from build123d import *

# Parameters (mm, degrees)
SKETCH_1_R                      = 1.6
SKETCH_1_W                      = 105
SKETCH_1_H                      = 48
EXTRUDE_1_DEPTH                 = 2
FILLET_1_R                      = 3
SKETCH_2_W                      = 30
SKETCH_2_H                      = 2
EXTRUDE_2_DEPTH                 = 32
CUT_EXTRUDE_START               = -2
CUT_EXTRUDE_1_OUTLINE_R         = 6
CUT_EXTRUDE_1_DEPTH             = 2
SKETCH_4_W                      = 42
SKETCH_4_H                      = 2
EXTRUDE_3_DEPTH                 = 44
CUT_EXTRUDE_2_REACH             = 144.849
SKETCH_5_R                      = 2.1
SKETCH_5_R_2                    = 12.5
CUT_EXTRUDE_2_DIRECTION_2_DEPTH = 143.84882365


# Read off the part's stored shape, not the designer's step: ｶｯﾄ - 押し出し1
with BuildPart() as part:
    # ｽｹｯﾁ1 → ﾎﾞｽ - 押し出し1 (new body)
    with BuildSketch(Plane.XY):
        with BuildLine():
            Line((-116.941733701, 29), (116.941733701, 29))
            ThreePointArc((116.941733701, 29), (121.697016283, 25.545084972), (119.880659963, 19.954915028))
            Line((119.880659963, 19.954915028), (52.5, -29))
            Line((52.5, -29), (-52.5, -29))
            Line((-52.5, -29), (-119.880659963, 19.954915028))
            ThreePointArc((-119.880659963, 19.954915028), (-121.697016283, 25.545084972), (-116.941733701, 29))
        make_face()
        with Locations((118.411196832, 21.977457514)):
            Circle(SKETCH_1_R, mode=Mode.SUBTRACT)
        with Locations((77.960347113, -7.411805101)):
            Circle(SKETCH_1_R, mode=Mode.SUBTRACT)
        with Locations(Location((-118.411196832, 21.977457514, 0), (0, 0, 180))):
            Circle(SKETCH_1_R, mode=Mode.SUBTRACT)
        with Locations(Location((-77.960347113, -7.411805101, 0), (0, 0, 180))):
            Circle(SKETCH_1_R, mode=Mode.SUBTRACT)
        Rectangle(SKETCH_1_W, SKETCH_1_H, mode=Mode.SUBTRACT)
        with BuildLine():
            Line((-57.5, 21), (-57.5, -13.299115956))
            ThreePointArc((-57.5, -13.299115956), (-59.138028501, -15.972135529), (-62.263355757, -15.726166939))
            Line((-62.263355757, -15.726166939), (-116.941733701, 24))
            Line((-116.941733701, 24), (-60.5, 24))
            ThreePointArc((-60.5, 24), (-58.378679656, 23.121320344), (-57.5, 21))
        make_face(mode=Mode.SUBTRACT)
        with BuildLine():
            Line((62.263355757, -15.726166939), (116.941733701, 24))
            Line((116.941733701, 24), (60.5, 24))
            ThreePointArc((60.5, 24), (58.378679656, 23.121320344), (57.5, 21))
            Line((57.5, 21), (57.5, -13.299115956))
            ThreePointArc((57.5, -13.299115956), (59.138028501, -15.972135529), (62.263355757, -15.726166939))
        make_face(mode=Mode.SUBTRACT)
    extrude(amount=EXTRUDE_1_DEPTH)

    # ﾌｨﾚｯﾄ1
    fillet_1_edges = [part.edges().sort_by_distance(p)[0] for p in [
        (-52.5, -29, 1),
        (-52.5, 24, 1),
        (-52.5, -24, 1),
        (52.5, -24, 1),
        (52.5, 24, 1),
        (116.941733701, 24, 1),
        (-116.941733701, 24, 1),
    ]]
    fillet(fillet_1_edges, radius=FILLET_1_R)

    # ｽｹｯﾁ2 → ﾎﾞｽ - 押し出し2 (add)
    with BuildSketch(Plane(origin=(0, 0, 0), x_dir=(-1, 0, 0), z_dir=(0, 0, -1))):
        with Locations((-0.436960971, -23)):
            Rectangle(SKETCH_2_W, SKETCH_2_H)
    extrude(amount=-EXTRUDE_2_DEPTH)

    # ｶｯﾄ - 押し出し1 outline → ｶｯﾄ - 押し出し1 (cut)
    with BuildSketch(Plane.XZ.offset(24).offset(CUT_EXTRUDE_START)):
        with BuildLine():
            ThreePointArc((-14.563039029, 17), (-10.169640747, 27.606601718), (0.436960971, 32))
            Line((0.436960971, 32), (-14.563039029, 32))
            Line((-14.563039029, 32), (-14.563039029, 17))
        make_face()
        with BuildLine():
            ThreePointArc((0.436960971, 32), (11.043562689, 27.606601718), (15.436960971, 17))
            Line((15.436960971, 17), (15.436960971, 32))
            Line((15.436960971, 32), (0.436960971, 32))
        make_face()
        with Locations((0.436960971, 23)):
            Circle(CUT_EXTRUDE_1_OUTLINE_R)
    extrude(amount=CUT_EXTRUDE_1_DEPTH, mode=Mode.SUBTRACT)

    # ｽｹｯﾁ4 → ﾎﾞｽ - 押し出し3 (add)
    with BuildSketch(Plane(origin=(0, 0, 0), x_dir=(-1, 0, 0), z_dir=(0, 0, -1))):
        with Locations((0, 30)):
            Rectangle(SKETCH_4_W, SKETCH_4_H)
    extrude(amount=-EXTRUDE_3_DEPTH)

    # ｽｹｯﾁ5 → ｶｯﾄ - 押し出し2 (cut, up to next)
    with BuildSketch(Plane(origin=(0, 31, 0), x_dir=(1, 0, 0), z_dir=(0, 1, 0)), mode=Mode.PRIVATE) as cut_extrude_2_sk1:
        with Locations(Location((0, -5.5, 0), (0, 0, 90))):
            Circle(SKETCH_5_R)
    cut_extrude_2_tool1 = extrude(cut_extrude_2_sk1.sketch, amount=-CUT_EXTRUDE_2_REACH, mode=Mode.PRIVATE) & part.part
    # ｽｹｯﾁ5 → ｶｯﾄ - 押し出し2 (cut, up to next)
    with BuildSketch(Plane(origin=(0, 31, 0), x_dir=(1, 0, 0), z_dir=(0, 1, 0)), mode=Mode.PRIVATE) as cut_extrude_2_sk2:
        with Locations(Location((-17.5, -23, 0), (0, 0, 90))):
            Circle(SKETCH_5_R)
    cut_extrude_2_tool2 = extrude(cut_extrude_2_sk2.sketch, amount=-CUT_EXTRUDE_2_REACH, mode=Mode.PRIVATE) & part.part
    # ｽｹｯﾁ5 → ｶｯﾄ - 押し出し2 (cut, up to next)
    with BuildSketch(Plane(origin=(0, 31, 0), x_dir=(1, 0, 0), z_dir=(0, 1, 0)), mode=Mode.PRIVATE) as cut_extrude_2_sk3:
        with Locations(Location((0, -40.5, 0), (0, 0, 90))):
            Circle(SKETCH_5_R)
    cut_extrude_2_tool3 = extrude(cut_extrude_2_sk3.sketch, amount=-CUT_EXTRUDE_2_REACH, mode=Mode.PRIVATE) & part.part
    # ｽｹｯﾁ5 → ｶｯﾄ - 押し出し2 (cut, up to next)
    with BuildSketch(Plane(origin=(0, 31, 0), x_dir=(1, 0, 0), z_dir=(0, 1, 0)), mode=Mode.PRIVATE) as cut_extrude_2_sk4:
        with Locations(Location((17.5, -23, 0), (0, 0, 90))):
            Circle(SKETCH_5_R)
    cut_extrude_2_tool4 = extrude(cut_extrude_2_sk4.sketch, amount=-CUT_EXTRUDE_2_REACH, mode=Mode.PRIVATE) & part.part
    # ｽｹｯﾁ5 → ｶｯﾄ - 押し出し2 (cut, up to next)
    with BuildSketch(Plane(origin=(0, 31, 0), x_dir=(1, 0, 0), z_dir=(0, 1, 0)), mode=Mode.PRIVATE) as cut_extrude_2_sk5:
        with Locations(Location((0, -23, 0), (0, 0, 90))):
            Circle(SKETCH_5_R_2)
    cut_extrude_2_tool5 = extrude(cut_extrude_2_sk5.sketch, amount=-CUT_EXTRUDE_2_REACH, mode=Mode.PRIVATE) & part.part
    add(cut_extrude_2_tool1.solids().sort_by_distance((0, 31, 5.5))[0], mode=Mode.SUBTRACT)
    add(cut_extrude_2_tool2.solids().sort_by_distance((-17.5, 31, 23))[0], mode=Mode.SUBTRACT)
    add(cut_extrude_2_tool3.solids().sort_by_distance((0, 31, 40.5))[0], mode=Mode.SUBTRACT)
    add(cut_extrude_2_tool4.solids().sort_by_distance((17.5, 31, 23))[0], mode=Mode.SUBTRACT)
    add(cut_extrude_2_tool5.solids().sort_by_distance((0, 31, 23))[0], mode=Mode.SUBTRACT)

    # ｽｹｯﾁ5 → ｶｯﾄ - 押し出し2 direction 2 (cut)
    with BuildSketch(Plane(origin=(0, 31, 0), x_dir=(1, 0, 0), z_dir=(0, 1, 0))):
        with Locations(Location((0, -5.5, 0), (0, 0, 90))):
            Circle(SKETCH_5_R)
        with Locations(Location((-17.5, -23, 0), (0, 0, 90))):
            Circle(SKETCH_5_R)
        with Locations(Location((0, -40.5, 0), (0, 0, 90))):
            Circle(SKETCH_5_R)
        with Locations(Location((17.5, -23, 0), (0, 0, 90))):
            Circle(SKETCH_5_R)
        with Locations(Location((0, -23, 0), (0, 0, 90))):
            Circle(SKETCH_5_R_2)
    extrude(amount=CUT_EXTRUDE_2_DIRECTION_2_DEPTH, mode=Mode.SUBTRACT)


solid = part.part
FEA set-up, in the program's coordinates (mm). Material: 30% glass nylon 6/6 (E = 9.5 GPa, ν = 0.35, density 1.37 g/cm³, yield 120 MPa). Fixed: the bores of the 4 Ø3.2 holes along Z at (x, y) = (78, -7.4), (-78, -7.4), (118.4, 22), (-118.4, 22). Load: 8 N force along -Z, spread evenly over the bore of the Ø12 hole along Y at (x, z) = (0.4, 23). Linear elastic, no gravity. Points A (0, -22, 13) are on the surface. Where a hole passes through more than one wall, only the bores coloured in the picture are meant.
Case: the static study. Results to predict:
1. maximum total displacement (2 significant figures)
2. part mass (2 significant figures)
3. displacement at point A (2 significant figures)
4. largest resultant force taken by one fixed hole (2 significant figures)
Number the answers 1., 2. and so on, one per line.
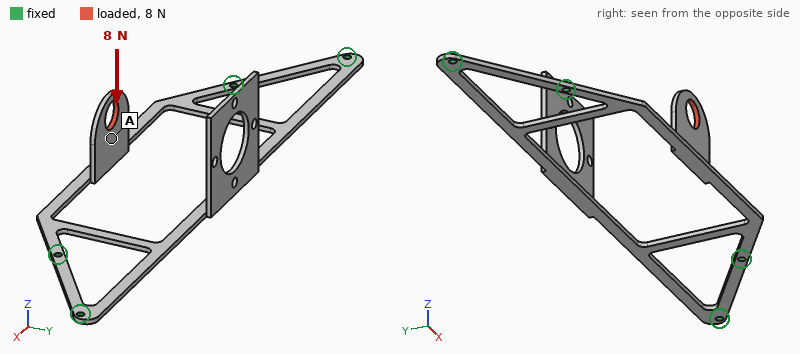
1. 2.9 mm
2. 14 g
3. 2.8 mm
4. 4.3 N
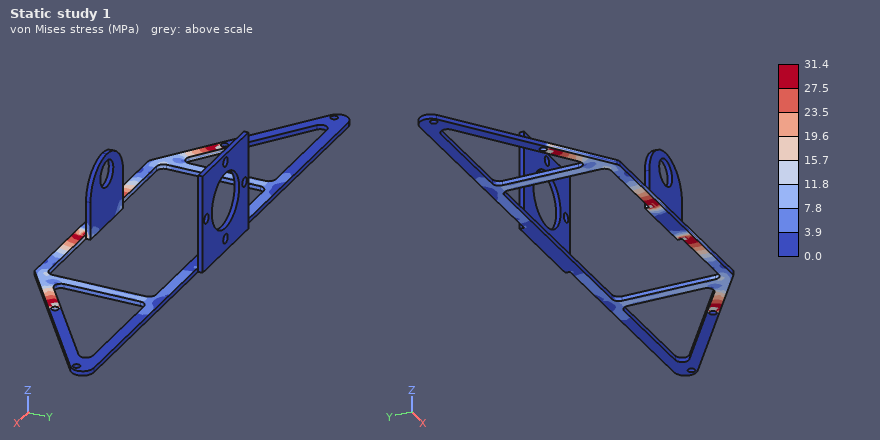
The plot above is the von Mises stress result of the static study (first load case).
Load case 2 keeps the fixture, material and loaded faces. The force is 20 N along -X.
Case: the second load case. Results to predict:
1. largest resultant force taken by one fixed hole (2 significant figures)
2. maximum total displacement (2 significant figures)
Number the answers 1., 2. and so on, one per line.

1. 12 N
2. 2.2 mm
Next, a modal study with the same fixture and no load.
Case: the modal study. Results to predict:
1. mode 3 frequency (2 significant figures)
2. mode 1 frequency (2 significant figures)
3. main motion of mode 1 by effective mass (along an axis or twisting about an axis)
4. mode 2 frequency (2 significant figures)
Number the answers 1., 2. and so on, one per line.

1. 160 Hz
2. 82 Hz
3. along Z
4. 130 Hz
